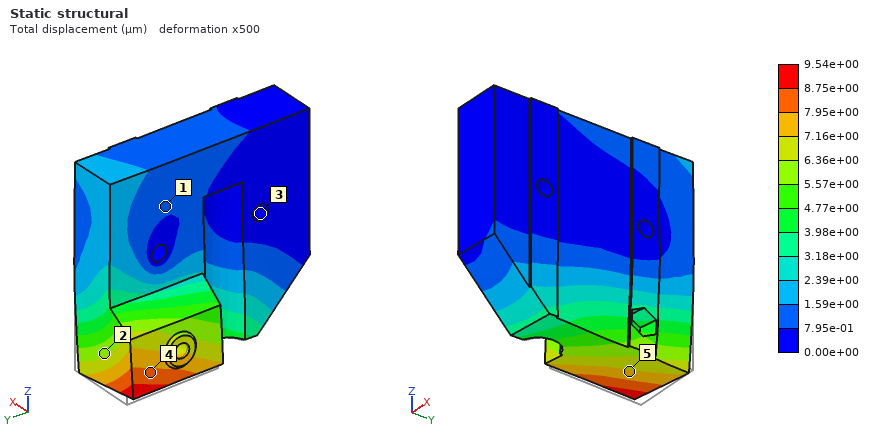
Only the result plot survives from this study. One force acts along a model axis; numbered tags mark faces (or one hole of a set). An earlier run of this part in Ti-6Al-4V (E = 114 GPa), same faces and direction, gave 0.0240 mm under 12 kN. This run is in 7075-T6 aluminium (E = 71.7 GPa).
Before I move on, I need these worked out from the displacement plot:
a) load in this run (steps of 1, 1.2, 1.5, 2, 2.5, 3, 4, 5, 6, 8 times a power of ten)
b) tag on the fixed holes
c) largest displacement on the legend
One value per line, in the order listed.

3 kN
3
9.54e+00 µm
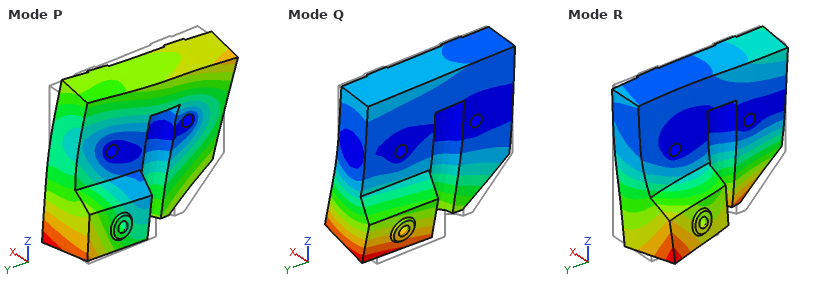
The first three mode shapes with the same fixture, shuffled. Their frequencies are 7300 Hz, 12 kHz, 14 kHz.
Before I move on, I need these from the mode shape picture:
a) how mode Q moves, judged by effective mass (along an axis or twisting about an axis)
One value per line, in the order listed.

along X
